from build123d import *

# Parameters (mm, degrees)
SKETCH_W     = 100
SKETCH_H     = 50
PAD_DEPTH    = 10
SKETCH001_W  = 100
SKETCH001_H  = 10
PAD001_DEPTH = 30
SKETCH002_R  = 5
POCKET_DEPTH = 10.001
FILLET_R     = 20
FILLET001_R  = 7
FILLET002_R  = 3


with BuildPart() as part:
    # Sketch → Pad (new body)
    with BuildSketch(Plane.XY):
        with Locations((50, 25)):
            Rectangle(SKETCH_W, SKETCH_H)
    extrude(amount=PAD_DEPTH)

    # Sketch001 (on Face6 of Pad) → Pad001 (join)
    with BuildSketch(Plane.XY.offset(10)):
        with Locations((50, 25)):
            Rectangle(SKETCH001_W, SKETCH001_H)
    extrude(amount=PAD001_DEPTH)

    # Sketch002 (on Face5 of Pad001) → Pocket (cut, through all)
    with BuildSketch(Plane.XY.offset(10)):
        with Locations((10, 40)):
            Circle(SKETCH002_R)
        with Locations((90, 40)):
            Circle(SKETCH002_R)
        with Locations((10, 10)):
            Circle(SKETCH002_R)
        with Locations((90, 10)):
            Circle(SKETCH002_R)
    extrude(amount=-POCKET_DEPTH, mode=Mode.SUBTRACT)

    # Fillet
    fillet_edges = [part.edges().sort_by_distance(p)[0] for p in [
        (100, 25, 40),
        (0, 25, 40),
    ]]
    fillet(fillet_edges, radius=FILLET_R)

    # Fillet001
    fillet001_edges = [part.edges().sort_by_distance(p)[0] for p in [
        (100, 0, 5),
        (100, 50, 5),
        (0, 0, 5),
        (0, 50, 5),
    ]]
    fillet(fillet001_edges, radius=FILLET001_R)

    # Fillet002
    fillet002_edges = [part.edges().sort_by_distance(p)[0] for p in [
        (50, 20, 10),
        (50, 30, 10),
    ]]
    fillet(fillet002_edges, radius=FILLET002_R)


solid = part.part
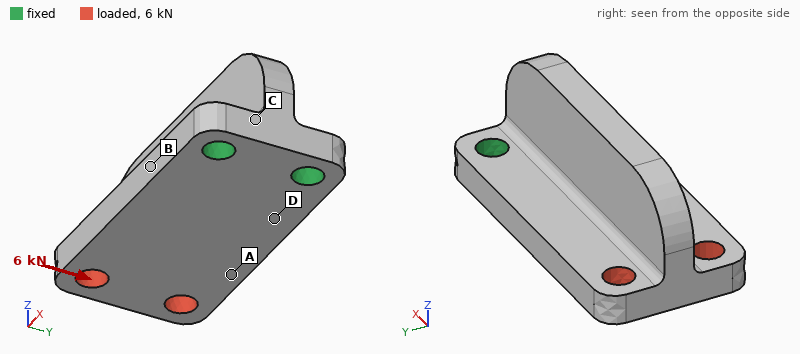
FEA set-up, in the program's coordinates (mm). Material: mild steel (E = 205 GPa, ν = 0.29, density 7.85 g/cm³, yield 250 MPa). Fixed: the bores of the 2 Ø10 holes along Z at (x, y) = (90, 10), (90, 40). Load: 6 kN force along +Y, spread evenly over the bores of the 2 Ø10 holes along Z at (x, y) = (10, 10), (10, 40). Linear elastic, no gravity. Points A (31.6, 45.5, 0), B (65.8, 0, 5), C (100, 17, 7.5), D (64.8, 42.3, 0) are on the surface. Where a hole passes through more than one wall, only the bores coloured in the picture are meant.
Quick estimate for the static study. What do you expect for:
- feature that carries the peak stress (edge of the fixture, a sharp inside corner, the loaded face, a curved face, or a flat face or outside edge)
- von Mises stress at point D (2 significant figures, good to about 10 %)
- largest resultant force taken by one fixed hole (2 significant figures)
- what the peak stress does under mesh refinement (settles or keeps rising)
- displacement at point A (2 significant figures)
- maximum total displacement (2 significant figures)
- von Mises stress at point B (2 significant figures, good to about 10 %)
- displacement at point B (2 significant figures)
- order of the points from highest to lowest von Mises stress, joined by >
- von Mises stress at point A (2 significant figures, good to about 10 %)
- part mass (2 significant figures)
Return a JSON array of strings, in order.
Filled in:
["edge of the fixture", "56 MPa", "14 kN", "keeps rising", "40 µm", "71 µm", "76 MPa", "15 µm", "B > D > A > C", "28 MPa", "590 g"]
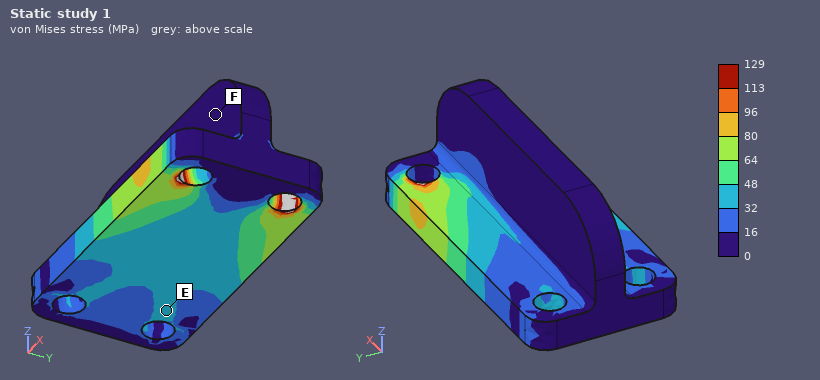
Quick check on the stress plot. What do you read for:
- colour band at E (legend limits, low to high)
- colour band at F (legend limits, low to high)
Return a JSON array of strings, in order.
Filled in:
["32 to 48 MPa", "0 to 16 MPa"]
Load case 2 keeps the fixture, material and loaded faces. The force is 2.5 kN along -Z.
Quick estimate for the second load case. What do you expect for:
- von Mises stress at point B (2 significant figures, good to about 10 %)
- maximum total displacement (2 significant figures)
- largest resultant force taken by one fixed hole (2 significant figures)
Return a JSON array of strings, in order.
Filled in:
["22 MPa", "0.15 mm", "1.3 kN"]
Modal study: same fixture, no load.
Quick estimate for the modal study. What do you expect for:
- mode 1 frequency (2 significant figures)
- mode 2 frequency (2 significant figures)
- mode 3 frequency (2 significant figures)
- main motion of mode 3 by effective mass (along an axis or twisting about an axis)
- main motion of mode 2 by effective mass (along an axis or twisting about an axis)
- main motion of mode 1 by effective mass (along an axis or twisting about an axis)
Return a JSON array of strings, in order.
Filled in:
["1500 Hz", "3100 Hz", "4400 Hz", "along Y", "along Y", "along Z"]
